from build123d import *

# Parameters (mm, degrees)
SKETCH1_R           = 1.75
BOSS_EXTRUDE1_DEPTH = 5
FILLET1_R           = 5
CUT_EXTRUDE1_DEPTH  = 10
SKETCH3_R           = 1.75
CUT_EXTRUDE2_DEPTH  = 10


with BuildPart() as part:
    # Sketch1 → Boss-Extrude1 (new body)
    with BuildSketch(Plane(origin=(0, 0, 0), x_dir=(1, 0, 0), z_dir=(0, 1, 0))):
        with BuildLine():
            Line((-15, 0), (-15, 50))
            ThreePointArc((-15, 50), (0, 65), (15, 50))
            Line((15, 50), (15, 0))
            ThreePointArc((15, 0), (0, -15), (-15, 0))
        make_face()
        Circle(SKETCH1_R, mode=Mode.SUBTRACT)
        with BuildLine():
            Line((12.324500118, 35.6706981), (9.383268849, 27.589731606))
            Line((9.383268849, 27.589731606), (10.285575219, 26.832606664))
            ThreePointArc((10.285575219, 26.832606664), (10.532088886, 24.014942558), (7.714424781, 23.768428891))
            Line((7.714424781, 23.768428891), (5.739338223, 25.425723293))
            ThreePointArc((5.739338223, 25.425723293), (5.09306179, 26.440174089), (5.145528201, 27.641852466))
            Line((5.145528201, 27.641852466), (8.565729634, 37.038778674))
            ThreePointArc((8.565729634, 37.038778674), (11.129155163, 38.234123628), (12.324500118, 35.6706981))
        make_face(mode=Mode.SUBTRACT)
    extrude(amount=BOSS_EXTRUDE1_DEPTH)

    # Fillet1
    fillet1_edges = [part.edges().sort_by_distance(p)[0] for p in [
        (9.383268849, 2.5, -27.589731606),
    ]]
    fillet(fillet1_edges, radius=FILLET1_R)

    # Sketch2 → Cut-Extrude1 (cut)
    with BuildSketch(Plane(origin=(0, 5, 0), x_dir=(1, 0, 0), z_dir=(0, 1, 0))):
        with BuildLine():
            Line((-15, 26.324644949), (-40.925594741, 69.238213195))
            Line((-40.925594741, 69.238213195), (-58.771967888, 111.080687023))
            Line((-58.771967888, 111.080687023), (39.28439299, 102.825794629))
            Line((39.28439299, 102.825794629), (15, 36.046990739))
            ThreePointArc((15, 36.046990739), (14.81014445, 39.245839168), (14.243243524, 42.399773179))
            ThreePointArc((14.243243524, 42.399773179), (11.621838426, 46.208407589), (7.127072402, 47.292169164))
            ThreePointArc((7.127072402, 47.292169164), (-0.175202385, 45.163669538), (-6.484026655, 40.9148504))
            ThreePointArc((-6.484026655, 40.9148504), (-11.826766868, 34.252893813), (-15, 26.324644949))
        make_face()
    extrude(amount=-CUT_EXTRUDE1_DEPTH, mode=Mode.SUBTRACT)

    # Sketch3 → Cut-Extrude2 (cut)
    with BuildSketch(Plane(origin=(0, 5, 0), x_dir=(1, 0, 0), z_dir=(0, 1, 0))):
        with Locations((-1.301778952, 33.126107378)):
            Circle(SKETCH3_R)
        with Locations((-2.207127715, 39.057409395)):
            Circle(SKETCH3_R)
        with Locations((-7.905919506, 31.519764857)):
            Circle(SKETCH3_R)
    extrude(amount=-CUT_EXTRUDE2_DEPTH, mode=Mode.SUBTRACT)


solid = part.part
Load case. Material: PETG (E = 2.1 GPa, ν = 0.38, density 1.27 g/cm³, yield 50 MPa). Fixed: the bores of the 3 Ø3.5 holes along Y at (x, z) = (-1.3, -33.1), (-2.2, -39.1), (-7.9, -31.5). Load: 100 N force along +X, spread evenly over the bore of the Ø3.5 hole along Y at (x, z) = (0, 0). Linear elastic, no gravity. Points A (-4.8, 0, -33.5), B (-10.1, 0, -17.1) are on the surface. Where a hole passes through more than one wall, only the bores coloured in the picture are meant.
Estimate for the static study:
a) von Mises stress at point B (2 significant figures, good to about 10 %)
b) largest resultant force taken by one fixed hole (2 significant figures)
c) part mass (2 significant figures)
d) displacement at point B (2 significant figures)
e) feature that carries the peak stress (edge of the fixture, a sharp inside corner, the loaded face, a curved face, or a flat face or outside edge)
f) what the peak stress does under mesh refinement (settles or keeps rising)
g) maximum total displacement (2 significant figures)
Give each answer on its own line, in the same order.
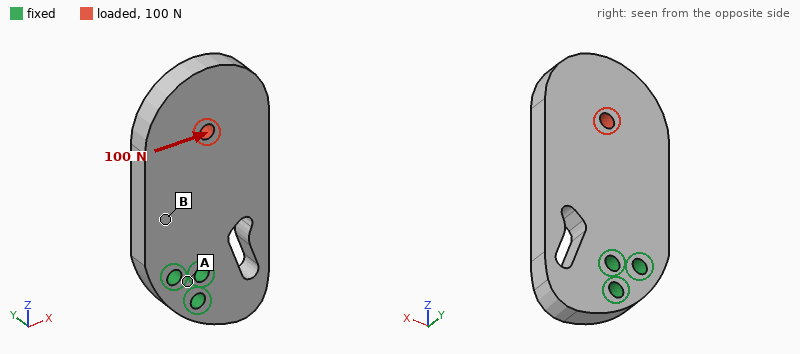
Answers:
2.3 MPa
260 N
9.7 g
0.087 mm
edge of the fixture
keeps rising
0.29 mm
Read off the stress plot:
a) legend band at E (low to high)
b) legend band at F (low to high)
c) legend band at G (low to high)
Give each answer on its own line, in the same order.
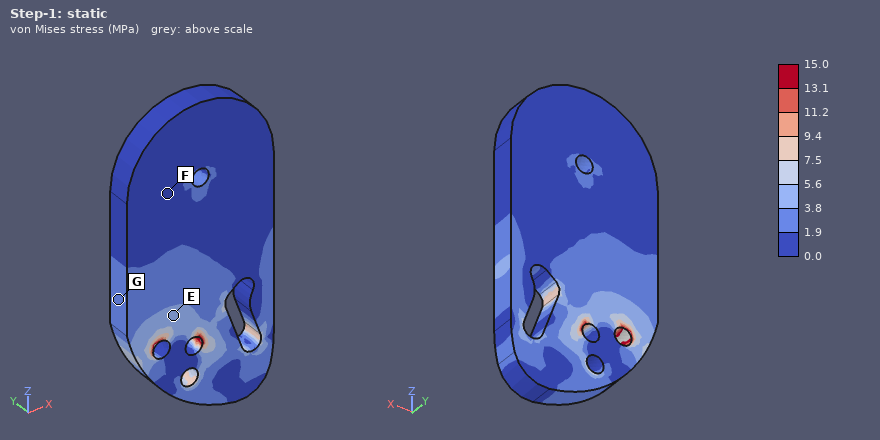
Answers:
3.8 to 5.6 MPa
0.0 to 1.9 MPa
1.9 to 3.8 MPa
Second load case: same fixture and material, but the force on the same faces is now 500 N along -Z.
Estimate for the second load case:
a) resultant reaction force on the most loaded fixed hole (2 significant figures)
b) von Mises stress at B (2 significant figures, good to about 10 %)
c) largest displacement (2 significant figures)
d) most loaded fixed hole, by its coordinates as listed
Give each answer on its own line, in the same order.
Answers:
370 N
2.9 MPa
0.20 mm
(-1.3, -33.1)
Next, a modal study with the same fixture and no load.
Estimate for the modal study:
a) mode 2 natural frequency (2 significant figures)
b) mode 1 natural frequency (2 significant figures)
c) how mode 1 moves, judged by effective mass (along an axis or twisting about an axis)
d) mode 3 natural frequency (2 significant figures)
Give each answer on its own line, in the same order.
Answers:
1400 Hz
490 Hz
along Y
1500 Hz
